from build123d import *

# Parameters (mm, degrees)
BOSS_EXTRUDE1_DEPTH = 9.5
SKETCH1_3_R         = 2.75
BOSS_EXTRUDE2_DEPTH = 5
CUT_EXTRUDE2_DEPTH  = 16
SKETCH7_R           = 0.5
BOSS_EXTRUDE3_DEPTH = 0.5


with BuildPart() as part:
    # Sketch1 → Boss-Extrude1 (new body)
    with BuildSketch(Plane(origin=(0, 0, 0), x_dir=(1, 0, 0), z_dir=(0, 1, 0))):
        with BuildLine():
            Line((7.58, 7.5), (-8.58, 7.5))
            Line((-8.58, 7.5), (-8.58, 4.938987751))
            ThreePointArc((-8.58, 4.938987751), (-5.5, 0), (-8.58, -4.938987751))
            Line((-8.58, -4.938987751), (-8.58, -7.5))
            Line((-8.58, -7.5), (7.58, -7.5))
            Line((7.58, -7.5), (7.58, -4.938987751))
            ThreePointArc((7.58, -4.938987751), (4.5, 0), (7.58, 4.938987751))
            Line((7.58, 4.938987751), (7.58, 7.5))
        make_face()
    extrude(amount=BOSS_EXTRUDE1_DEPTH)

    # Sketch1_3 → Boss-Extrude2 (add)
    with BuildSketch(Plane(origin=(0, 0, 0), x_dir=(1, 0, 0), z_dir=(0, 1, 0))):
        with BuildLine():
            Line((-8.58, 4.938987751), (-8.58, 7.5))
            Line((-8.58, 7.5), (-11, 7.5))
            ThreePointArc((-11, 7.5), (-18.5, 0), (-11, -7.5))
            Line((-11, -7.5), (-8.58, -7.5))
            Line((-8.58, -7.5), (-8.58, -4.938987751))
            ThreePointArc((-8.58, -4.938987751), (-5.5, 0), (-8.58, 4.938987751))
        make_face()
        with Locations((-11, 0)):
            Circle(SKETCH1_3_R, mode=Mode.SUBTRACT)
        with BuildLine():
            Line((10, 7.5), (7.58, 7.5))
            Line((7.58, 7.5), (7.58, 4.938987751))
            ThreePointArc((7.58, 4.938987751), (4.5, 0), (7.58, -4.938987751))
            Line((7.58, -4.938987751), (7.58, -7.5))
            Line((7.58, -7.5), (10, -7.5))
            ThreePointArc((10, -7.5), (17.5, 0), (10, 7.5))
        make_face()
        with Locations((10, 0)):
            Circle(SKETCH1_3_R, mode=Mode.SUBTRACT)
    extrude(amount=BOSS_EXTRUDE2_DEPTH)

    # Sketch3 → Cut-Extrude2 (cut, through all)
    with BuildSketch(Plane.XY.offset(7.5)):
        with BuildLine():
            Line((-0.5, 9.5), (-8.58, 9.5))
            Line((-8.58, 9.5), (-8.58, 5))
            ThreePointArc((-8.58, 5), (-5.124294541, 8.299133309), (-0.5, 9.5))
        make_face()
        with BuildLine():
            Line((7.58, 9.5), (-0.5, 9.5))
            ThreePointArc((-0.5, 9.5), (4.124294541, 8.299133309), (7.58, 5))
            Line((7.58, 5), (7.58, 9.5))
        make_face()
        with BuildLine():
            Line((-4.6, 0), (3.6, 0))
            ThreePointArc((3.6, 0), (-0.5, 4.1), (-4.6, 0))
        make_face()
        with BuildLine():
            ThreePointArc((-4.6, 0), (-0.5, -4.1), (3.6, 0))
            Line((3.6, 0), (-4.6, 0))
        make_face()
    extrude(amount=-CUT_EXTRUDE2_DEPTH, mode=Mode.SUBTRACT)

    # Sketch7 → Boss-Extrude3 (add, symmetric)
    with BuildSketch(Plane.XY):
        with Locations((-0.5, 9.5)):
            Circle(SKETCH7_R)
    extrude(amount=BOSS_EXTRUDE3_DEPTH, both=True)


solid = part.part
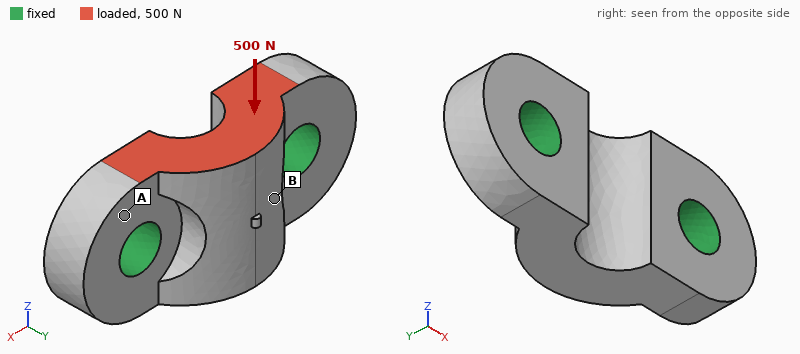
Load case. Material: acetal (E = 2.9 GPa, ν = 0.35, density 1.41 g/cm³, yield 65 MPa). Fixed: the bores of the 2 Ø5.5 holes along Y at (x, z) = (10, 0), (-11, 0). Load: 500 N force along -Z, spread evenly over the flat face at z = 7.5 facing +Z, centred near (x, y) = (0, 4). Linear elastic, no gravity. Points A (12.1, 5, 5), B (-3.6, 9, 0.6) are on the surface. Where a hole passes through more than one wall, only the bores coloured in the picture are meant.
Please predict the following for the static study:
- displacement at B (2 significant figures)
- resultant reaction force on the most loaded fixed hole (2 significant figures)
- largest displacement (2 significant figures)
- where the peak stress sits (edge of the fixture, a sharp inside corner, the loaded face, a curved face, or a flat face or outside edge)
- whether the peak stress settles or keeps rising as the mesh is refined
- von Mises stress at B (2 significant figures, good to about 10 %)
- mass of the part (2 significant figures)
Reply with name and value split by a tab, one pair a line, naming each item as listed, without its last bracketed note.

displacement at B	44 µm
resultant reaction force on the most loaded fixed hole	250 N
largest displacement	67 µm
where the peak stress sits	edge of the fixture
whether the peak stress settles or keeps rising as the mesh is refined	keeps rising
von Mises stress at B	4.2 MPa
mass of the part	3.6 g
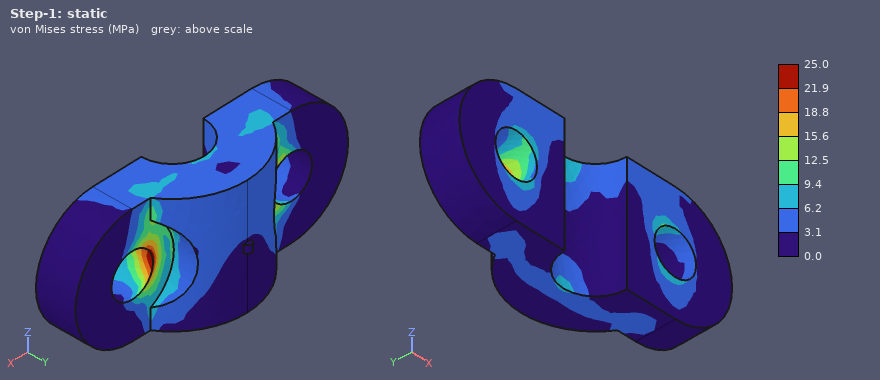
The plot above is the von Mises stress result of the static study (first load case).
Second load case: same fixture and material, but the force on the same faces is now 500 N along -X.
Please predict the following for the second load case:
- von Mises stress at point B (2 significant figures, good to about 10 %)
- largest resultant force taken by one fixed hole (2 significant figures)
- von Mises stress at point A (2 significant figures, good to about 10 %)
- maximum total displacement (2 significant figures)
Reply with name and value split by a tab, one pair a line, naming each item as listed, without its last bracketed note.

von Mises stress at point B	2.1 MPa
largest resultant force taken by one fixed hole	280 N
von Mises stress at point A	5.0 MPa
maximum total displacement	42 µm
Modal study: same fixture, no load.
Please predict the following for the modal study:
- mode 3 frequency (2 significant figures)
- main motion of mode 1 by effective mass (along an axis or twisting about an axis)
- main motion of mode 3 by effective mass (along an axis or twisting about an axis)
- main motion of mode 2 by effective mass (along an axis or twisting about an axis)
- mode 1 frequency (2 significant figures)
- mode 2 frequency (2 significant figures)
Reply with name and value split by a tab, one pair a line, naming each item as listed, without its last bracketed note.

mode 3 frequency	20 kHz
main motion of mode 1 by effective mass	along Z
main motion of mode 3 by effective mass	along Z
main motion of mode 2 by effective mass	along Y
mode 1 frequency	10 kHz
mode 2 frequency	15 kHz
